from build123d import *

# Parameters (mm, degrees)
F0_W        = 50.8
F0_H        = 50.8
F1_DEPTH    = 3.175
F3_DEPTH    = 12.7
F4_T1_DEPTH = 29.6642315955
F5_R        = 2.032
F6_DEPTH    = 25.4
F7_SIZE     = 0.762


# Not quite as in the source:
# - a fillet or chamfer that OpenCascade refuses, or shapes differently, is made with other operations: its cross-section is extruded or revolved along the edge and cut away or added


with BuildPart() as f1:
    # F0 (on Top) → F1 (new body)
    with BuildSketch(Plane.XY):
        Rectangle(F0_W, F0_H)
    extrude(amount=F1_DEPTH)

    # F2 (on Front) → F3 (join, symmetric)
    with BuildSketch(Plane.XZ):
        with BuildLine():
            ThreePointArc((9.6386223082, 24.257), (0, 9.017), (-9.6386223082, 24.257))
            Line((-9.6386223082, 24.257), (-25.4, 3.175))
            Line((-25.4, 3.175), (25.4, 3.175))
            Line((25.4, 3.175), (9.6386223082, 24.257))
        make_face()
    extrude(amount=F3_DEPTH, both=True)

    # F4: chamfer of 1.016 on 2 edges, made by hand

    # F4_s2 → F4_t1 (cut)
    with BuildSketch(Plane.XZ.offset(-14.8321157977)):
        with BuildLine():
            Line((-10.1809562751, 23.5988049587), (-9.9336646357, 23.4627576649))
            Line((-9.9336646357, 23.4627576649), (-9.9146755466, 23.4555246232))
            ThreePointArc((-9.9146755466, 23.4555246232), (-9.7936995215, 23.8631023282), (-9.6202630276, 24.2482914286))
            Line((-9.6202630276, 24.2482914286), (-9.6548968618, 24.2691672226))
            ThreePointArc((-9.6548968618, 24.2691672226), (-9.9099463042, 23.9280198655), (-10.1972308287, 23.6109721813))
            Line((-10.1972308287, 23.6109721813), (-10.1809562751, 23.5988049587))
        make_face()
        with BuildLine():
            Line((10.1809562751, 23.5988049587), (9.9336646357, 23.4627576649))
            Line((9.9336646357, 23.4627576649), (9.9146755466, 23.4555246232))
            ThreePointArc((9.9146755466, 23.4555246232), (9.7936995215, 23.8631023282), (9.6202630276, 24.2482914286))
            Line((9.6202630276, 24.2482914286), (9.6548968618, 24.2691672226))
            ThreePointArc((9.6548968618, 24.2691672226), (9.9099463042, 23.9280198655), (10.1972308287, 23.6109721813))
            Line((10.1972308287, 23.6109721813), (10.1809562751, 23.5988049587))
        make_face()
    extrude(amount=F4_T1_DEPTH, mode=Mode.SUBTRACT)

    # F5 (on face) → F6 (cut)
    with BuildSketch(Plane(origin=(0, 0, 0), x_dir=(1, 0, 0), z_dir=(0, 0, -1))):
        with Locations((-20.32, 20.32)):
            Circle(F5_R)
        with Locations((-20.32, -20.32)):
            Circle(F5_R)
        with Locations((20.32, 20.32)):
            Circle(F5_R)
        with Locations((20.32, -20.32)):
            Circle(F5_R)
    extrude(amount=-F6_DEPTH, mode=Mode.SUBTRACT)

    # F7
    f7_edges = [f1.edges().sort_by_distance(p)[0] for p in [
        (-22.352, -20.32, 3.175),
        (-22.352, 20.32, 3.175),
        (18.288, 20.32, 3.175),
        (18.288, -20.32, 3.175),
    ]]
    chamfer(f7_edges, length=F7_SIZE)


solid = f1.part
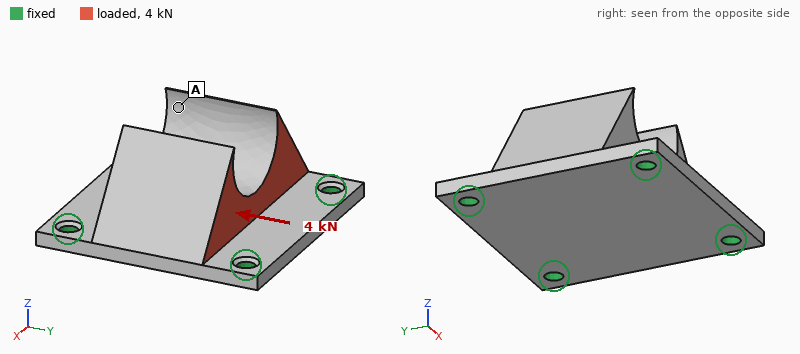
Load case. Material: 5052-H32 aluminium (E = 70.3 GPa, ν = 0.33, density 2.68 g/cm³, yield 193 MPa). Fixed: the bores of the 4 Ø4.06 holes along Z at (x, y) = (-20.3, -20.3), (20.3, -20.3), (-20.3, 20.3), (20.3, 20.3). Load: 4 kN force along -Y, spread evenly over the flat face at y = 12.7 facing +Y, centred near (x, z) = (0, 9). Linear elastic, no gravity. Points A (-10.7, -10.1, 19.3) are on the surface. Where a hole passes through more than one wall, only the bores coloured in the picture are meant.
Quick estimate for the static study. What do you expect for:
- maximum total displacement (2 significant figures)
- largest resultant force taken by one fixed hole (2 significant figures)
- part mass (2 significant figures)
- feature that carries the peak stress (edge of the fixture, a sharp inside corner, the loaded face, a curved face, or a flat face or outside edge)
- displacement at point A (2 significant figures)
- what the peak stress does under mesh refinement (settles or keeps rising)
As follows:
25 µm
1.2 kN
53 g
edge of the fixture
19 µm
keeps rising
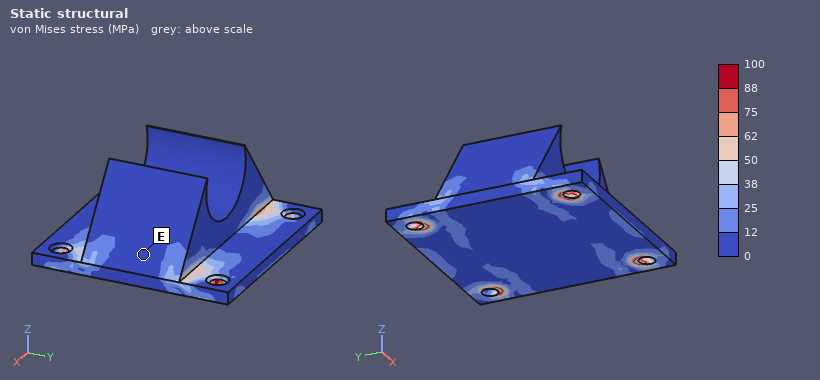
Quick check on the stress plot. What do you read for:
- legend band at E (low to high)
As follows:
0 to 12 MPa
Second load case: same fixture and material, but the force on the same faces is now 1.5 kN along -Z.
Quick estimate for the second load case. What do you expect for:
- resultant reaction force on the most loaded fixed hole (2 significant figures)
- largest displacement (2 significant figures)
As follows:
700 N
27 µm
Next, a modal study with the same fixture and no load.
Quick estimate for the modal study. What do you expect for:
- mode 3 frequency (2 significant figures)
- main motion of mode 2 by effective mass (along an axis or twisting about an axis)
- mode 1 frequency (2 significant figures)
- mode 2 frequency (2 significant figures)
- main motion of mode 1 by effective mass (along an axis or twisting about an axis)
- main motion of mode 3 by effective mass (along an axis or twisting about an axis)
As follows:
12 kHz
along X
7600 Hz
10 kHz
along Z
along Y
